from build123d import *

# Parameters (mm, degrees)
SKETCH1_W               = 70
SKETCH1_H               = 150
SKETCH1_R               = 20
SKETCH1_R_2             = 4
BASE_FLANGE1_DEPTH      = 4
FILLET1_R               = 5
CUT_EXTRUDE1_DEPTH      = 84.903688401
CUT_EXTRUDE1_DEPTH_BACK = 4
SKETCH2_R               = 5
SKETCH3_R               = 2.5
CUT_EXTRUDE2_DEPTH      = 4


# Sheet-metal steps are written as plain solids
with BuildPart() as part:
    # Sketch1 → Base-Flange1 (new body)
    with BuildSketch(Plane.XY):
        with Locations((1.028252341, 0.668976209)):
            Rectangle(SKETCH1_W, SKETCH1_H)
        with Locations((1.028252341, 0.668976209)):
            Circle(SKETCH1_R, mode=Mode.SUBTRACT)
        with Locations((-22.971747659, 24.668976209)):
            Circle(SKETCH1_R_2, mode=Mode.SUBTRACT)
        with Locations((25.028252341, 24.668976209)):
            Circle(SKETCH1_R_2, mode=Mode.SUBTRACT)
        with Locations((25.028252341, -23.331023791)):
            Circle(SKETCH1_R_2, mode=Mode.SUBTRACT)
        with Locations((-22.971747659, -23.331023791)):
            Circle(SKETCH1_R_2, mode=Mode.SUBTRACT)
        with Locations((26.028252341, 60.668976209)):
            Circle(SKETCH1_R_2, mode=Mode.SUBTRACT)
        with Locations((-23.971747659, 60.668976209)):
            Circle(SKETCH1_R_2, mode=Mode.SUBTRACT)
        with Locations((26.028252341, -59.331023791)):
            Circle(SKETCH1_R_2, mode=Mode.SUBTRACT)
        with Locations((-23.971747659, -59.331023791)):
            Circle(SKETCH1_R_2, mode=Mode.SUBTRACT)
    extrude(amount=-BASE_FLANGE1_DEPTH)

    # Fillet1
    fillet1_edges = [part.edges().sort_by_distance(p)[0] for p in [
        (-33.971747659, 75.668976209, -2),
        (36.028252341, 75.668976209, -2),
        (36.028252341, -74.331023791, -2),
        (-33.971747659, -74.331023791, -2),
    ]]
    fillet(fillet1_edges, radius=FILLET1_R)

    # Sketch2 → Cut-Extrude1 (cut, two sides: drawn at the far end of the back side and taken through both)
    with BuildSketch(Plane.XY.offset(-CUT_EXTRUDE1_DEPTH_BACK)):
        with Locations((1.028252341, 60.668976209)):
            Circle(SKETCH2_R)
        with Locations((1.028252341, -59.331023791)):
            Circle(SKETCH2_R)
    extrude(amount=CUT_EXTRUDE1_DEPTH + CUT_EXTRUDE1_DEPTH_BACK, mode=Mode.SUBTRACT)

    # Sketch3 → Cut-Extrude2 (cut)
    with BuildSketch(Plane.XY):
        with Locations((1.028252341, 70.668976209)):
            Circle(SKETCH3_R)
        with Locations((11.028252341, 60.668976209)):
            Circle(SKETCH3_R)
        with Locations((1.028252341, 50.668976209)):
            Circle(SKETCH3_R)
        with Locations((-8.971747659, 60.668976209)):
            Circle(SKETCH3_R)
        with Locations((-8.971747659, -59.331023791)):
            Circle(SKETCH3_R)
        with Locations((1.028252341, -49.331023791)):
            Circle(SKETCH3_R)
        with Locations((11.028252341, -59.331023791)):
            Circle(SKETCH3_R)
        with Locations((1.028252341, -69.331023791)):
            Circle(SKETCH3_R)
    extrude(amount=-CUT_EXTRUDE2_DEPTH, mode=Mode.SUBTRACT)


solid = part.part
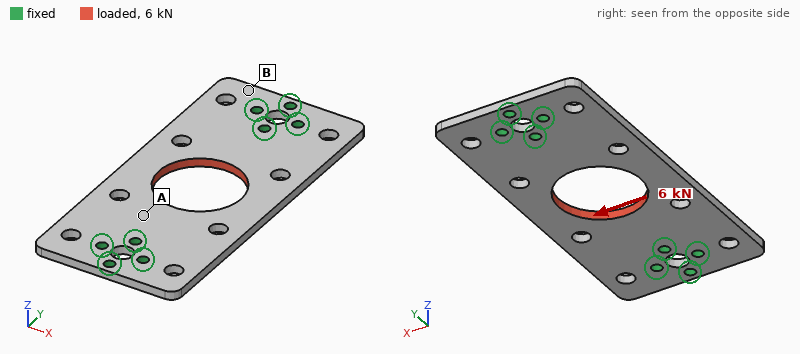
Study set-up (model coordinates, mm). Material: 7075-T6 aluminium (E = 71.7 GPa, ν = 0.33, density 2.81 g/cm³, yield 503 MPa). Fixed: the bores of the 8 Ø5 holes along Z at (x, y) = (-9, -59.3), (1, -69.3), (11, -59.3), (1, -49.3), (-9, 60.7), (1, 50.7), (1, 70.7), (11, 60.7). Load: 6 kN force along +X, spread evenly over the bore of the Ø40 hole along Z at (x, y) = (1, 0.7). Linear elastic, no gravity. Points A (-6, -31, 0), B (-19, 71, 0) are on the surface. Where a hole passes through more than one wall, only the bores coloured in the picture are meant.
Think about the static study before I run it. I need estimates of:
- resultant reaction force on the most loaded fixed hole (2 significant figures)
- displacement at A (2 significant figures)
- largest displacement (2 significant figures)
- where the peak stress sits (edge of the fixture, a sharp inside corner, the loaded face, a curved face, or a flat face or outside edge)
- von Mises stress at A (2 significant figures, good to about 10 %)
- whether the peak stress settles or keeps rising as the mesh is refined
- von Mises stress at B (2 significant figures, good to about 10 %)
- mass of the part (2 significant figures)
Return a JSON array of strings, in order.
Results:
["2.9 kN", "18 µm", "38 µm", "edge of the fixture", "29 MPa", "keeps rising", "6.0 MPa", "96 g"]
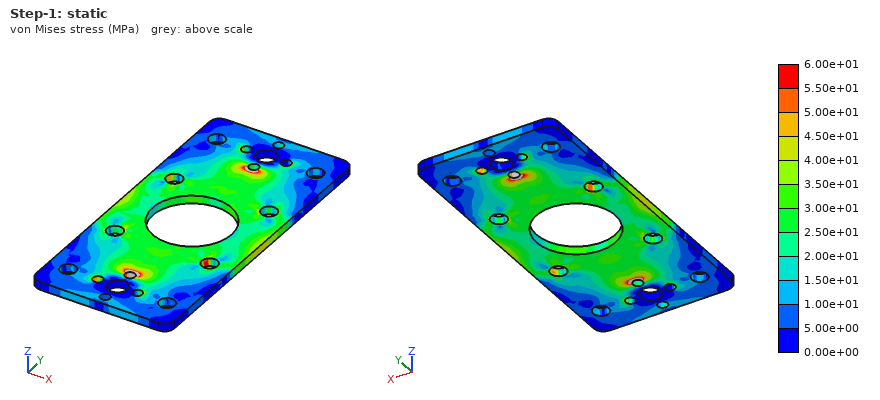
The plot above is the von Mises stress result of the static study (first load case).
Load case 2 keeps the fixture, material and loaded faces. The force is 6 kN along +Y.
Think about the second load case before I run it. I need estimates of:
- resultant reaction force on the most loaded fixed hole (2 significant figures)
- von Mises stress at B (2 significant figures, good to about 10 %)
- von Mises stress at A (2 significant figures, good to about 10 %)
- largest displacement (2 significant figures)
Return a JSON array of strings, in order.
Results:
["1.2 kN", "3.2 MPa", "18 MPa", "13 µm"]
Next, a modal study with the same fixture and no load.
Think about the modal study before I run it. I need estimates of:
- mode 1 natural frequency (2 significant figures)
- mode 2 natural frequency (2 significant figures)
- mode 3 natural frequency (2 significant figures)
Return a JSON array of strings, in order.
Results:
["1800 Hz", "1800 Hz", "3700 Hz"]
